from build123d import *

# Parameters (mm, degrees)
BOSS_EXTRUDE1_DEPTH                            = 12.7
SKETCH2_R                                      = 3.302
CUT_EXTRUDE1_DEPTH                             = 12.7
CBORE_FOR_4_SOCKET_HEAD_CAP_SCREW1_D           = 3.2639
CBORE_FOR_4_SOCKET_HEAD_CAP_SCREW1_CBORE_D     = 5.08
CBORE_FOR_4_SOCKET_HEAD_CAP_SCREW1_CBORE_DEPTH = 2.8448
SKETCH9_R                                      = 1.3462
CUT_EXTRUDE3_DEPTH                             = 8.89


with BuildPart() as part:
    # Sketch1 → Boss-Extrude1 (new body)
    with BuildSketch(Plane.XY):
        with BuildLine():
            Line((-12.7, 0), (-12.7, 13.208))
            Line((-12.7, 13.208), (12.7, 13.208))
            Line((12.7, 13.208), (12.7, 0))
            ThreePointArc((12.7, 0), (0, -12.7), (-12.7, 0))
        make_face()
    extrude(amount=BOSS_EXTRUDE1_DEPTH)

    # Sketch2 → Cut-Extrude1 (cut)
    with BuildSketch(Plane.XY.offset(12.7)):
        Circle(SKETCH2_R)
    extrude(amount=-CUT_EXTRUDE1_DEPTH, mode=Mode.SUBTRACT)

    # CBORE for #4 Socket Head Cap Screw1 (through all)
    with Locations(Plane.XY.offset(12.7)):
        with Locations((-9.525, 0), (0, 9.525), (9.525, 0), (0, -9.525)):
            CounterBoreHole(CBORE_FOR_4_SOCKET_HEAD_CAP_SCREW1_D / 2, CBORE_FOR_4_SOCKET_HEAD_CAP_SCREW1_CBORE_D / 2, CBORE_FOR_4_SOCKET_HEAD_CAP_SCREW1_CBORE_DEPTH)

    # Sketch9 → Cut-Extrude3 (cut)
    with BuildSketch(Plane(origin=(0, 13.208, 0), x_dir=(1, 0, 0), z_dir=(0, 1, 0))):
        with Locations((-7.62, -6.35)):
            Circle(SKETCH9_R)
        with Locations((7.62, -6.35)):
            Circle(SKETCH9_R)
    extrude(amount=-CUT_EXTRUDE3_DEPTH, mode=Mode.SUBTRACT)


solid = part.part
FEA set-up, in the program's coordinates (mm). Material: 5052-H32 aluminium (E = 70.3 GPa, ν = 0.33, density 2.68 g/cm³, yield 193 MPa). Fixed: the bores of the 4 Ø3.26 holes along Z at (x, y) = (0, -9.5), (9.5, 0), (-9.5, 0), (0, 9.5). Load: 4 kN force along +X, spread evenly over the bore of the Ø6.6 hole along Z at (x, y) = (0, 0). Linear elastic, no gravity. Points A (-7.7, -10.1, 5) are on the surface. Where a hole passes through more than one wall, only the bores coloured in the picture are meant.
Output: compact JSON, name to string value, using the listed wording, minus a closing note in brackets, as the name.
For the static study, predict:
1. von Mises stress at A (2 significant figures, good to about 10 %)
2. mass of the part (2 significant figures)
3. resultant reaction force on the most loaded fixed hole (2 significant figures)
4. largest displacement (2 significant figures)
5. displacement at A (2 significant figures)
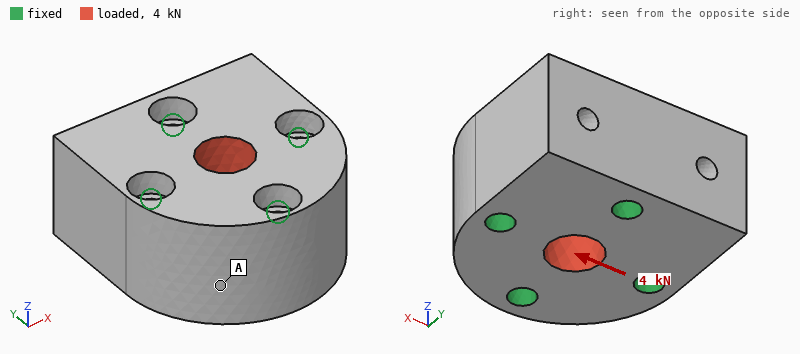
{"von Mises stress at A": "5.1 MPa", "mass of the part": "17 g", "resultant reaction force on the most loaded fixed hole": "1.3 kN", "largest displacement": "2.5 µm", "displacement at A": "0.55 µm"}
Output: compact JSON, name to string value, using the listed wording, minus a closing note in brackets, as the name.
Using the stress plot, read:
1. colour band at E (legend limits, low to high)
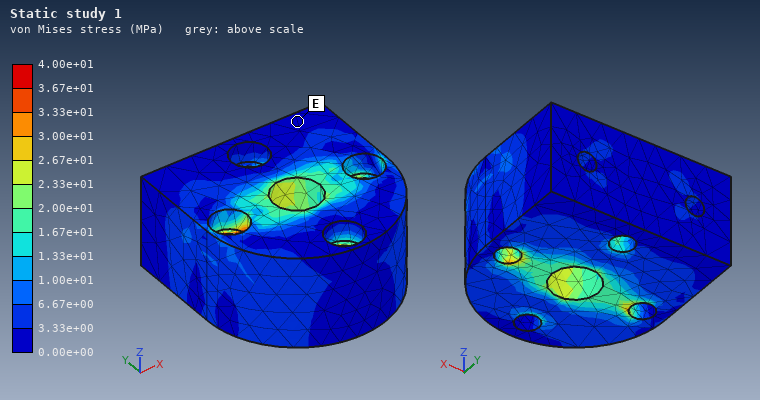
{"colour band at E": "0.00e+00 to 3.33e+00 MPa"}
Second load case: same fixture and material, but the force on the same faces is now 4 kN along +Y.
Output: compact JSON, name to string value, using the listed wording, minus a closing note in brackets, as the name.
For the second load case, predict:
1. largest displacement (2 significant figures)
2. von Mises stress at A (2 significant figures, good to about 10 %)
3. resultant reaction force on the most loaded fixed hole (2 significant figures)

{"largest displacement": "2.4 µm", "von Mises stress at A": "5.7 MPa", "resultant reaction force on the most loaded fixed hole": "1.3 kN"}
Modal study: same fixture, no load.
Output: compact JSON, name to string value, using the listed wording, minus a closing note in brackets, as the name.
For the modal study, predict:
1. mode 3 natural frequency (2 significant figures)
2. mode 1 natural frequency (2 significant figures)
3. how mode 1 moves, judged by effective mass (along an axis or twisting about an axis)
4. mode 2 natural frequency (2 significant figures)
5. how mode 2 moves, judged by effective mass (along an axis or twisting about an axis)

{"mode 3 natural frequency": "81 kHz", "mode 1 natural frequency": "54 kHz", "how mode 1 moves, judged by effective mass": "twisting about Y", "mode 2 natural frequency": "57 kHz", "how mode 2 moves, judged by effective mass": "along Z"}
